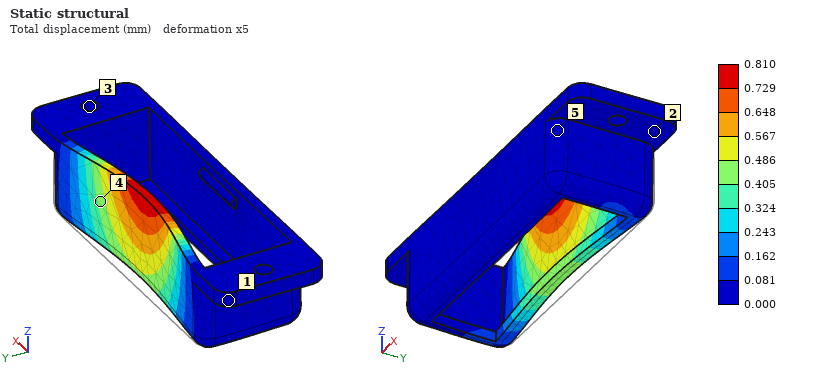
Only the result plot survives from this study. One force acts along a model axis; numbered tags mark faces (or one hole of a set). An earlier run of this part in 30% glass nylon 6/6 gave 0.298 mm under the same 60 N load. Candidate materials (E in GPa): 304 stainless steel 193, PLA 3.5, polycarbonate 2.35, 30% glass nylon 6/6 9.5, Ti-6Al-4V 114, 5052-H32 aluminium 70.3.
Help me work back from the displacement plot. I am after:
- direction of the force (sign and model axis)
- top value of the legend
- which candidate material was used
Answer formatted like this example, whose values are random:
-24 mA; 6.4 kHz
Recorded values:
-Y; 0.810 mm; PLA
